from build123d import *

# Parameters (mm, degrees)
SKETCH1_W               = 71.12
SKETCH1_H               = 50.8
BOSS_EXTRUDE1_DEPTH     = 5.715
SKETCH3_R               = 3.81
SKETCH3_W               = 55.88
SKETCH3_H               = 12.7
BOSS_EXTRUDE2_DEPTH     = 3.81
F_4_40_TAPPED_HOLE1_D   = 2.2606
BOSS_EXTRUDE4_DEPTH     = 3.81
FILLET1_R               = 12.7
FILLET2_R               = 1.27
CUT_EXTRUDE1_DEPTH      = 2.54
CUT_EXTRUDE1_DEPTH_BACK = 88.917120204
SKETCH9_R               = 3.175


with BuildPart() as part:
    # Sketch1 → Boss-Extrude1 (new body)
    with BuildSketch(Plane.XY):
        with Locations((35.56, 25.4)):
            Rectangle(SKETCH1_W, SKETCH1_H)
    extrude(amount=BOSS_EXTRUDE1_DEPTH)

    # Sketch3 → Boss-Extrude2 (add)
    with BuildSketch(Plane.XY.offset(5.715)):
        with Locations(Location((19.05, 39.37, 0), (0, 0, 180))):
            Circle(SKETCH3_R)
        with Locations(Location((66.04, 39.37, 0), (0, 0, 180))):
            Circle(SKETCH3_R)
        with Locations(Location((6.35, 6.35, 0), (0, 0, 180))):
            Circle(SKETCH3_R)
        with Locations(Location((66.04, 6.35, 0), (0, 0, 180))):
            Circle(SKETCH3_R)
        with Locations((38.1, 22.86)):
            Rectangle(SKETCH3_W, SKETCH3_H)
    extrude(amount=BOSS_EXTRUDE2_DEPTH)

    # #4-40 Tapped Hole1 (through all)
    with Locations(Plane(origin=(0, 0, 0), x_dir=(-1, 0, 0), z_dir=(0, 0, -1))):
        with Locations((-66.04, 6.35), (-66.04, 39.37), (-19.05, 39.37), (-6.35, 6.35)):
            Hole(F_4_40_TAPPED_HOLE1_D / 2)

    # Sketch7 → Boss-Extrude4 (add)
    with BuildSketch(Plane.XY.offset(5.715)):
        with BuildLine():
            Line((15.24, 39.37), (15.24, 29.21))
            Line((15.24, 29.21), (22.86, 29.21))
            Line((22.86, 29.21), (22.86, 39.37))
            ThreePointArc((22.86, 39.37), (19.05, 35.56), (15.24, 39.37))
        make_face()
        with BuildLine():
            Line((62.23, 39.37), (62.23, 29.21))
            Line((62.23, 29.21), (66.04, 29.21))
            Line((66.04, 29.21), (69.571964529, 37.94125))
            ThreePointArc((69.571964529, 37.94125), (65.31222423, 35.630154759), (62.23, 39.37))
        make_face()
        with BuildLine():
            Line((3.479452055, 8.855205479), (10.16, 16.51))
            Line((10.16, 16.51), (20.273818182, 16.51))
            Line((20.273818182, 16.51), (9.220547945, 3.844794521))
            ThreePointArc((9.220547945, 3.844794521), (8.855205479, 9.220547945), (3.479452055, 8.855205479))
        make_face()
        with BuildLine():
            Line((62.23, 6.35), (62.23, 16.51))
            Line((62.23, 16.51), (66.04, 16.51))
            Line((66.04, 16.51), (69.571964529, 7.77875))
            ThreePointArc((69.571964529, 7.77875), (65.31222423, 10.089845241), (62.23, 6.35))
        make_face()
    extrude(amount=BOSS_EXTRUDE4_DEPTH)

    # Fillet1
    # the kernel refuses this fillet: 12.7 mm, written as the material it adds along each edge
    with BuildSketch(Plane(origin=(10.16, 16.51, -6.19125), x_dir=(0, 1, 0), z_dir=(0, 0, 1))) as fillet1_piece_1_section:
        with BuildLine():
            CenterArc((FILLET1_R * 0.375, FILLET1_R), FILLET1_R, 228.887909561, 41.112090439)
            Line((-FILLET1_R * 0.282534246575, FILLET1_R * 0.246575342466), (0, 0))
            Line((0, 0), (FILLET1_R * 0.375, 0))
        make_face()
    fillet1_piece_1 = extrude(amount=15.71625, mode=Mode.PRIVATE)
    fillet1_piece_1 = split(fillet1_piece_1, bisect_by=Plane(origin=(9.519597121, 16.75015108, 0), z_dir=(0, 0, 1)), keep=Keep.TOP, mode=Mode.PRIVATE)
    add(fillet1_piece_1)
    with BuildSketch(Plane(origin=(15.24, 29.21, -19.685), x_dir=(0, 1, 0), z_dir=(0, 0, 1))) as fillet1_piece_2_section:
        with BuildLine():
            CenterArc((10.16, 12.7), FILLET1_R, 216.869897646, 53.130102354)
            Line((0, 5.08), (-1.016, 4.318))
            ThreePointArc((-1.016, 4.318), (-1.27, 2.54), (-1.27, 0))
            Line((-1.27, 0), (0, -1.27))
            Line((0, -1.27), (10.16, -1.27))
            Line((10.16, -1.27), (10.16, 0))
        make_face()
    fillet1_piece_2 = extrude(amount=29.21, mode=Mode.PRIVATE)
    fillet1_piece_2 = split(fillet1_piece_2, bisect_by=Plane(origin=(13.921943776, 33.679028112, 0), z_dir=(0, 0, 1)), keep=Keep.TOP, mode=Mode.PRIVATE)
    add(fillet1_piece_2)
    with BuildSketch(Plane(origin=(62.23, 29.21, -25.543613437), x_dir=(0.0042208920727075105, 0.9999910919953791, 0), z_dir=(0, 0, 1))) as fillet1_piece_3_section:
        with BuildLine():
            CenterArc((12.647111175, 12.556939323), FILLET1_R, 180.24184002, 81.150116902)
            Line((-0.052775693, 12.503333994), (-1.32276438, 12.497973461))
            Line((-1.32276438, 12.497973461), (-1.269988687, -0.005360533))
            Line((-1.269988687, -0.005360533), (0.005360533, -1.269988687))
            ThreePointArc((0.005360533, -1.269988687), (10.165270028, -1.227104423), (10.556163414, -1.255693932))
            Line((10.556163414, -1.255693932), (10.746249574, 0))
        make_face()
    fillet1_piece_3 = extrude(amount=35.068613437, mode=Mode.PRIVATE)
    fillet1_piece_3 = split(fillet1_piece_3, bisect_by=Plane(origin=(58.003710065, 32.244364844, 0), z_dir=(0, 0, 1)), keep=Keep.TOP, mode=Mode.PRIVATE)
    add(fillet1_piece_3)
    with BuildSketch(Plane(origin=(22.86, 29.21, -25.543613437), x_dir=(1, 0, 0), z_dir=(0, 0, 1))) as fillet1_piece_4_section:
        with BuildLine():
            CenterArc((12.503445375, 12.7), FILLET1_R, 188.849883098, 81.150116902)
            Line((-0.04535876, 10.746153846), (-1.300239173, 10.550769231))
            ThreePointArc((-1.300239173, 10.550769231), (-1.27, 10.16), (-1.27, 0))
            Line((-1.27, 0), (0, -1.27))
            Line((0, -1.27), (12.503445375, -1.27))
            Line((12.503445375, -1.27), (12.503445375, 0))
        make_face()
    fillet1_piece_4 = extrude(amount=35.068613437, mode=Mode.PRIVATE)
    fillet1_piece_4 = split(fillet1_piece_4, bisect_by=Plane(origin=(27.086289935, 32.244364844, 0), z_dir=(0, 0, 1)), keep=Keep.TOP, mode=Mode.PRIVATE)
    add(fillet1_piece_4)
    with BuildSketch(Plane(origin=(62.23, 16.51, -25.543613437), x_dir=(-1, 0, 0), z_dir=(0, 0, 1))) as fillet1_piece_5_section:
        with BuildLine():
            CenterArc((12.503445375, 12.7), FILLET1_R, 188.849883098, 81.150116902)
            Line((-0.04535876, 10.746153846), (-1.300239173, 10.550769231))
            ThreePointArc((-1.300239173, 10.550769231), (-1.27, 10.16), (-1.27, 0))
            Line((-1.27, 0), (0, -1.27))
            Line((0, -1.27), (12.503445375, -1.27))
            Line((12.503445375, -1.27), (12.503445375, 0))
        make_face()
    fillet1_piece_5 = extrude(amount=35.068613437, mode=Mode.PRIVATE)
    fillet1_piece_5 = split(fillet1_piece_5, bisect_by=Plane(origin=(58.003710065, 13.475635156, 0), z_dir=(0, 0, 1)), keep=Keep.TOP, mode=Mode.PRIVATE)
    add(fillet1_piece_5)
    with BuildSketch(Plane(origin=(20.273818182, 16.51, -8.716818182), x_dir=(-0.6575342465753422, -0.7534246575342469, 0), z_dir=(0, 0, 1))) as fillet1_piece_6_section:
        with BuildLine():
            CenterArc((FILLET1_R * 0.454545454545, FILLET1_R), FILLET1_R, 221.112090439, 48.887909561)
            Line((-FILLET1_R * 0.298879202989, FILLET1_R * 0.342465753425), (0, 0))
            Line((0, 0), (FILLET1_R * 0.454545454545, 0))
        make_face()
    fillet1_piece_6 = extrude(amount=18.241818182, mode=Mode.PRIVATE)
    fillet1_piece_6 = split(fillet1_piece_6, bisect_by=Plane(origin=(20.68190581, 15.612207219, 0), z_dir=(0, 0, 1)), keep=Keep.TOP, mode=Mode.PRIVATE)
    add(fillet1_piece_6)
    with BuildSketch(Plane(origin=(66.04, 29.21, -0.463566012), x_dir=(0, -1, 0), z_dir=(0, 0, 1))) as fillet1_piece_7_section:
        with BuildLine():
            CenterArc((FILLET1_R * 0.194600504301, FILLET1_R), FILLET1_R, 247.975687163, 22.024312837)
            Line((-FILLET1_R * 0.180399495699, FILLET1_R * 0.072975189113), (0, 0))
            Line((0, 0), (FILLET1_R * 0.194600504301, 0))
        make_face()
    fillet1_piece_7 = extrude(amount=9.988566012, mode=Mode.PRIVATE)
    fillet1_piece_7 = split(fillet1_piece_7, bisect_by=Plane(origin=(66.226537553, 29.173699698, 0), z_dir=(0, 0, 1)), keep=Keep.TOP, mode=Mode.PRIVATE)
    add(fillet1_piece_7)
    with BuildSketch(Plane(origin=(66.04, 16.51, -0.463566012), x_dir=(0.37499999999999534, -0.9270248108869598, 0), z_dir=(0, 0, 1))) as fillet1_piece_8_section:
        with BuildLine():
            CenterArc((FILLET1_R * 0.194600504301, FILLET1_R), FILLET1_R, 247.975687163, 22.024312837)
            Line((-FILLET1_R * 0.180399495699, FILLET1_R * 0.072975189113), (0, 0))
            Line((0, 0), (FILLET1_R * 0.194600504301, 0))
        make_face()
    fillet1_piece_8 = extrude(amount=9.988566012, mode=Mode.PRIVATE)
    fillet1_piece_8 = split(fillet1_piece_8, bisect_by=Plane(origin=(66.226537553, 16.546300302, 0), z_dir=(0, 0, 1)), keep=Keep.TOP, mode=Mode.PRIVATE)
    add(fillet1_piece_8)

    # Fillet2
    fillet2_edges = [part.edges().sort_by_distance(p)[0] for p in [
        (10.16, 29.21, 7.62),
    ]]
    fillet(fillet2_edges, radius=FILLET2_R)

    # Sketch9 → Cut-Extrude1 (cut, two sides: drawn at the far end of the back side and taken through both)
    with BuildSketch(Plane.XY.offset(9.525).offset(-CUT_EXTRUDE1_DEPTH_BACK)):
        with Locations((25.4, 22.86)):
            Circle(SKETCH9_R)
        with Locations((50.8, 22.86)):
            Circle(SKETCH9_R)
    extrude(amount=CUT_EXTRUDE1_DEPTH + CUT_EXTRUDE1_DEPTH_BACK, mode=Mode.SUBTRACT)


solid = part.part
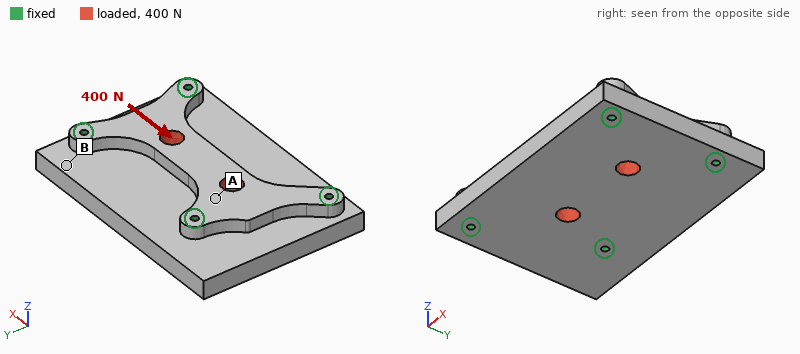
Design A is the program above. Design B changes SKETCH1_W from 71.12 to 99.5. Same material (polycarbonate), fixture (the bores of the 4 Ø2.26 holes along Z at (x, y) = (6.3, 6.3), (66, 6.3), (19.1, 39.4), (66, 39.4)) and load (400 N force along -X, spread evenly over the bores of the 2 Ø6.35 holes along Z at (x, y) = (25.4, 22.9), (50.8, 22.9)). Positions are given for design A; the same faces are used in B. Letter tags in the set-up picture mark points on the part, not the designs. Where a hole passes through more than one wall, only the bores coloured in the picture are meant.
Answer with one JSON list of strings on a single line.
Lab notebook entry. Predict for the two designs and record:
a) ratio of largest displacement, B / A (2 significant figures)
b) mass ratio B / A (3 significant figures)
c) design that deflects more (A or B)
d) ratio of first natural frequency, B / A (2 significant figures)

["0.91", "1.34", "A", "0.58"]
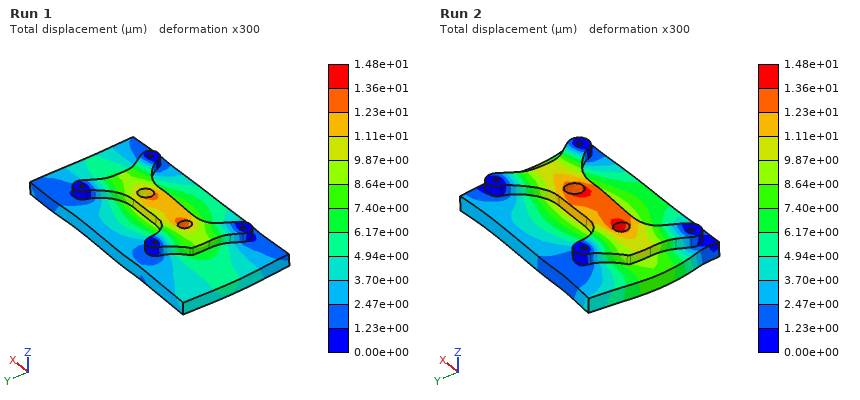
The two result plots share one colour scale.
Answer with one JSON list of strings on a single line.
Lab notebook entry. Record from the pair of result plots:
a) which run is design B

["Run 1"]
